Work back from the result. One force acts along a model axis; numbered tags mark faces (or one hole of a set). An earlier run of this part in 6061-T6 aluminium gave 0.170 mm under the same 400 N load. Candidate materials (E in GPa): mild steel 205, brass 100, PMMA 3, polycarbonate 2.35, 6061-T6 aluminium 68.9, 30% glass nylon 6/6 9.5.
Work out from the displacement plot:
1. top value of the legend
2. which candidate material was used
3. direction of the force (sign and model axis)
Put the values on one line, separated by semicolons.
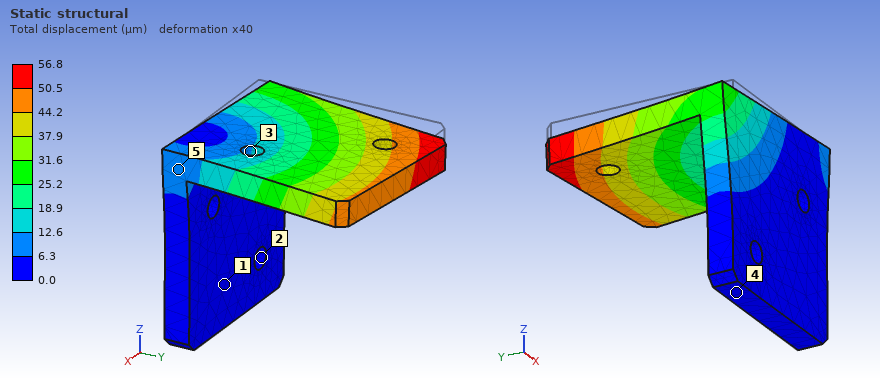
56.8 µm; mild steel; +X
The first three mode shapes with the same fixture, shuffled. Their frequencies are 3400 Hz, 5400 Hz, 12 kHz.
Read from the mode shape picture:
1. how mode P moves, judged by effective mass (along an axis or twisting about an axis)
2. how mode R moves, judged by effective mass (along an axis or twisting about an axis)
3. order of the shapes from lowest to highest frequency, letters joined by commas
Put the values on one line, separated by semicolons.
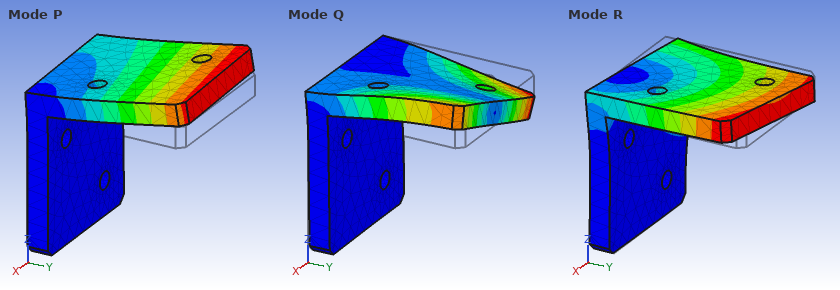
along Z; along X; P, R, Q
